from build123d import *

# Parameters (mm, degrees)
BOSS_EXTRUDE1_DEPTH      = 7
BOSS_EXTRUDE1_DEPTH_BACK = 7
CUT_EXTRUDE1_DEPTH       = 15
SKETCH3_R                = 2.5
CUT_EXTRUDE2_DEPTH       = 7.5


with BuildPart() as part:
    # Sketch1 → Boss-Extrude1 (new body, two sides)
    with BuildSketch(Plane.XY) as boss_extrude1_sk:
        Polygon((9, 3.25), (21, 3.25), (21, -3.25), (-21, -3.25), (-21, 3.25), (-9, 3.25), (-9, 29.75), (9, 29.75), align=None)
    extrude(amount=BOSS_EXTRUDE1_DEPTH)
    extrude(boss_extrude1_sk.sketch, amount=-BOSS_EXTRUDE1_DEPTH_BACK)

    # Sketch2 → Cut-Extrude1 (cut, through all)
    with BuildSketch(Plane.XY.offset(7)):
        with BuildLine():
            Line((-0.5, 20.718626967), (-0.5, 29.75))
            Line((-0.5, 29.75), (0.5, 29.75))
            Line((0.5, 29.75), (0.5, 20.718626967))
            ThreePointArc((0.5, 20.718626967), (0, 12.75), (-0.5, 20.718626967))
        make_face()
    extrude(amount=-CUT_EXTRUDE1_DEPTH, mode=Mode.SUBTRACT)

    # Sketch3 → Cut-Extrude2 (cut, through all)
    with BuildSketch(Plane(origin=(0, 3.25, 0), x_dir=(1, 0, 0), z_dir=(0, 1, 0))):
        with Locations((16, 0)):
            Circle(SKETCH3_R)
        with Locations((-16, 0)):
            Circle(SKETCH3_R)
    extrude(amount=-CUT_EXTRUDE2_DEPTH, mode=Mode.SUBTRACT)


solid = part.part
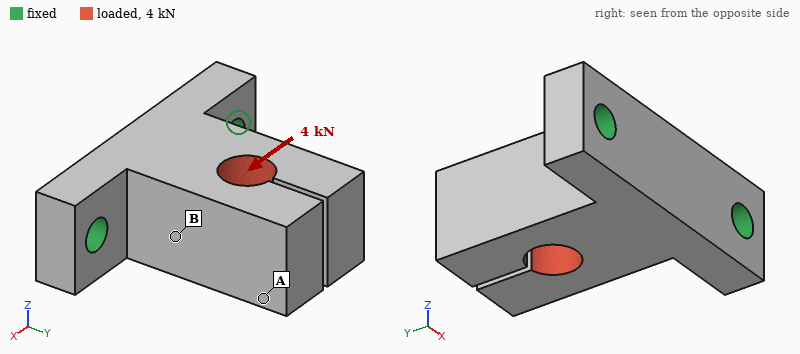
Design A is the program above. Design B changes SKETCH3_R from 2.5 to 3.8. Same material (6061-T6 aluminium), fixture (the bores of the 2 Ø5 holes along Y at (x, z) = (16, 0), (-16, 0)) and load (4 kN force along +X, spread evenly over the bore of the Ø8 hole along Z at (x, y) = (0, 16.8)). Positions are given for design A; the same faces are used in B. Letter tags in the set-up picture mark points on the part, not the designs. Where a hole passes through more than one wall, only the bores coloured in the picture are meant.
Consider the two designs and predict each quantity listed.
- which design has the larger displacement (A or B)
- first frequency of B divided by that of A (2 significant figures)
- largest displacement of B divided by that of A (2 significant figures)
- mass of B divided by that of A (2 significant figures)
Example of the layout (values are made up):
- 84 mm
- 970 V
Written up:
- A
- 1.1
- 0.91
- 0.96
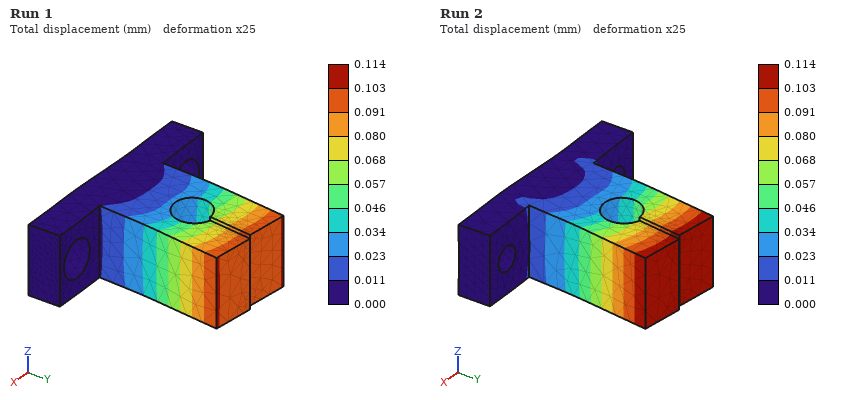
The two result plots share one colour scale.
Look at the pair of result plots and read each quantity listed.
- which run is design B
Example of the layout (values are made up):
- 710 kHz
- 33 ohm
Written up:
- Run 1
